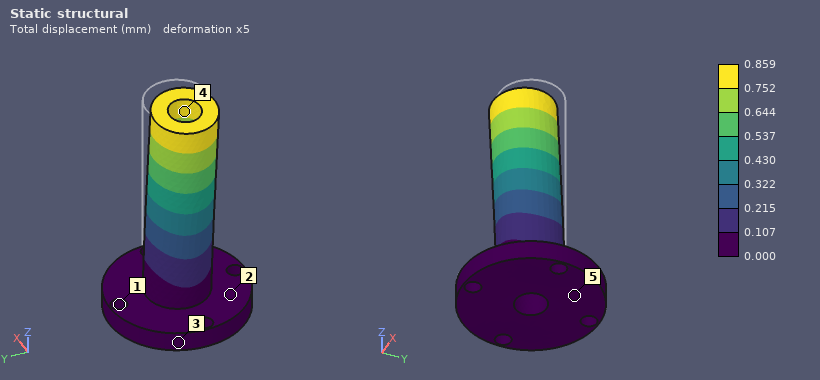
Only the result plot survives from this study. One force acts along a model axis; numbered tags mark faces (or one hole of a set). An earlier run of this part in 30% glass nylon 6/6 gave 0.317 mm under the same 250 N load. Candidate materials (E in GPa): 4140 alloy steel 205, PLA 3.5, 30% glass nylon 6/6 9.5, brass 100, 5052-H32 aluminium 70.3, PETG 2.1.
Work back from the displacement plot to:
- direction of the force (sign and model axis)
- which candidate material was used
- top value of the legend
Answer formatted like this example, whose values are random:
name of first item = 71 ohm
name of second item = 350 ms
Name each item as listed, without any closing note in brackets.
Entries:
direction of the force = -X
which candidate material was used = PLA
top value of the legend = 0.859 mm
